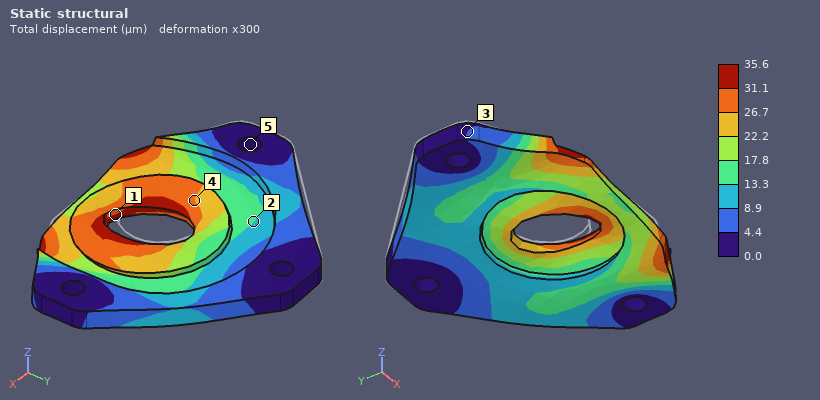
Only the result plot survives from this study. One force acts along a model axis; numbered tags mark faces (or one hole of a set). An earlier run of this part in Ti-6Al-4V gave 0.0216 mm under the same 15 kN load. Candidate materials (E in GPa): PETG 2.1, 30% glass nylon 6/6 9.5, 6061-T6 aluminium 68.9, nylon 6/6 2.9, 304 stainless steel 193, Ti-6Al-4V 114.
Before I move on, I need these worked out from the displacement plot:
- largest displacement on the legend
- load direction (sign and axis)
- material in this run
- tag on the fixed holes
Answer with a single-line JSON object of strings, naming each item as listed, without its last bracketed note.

{"largest displacement on the legend": "35.6 µm", "load direction": "+X", "material in this run": "6061-T6 aluminium", "tag on the fixed holes": "5"}
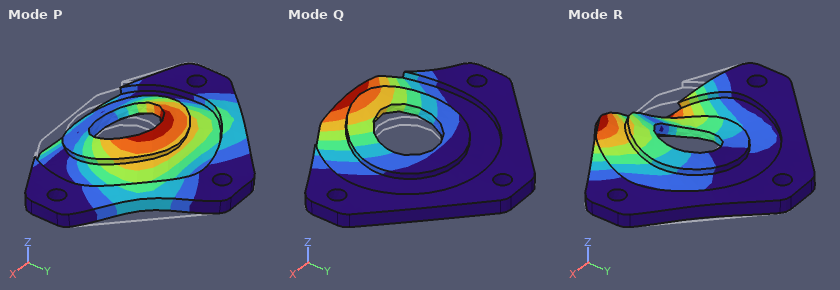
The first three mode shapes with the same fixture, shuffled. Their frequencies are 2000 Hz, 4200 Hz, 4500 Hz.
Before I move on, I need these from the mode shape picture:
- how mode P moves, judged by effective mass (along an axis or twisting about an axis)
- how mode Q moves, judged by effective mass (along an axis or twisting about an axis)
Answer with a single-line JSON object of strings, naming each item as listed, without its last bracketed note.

{"how mode P moves, judged by effective mass": "along Z", "how mode Q moves, judged by effective mass": "along Z"}
